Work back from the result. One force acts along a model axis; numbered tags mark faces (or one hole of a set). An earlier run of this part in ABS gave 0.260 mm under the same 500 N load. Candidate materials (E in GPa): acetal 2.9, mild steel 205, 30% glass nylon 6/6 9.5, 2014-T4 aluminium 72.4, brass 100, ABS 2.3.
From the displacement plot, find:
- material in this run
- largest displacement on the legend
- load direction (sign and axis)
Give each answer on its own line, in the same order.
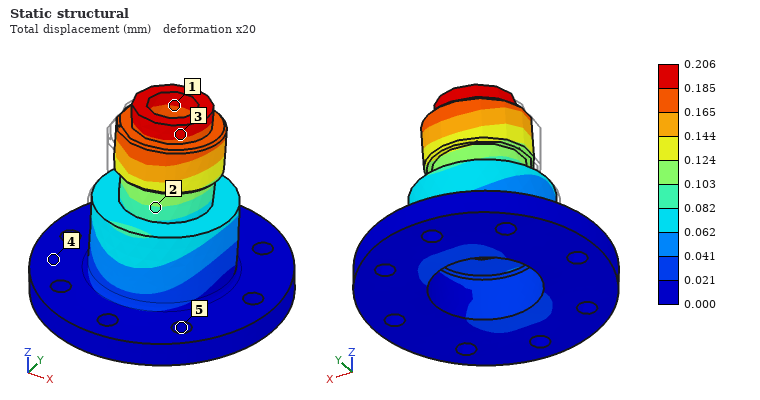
acetal
0.206 mm
+Y
